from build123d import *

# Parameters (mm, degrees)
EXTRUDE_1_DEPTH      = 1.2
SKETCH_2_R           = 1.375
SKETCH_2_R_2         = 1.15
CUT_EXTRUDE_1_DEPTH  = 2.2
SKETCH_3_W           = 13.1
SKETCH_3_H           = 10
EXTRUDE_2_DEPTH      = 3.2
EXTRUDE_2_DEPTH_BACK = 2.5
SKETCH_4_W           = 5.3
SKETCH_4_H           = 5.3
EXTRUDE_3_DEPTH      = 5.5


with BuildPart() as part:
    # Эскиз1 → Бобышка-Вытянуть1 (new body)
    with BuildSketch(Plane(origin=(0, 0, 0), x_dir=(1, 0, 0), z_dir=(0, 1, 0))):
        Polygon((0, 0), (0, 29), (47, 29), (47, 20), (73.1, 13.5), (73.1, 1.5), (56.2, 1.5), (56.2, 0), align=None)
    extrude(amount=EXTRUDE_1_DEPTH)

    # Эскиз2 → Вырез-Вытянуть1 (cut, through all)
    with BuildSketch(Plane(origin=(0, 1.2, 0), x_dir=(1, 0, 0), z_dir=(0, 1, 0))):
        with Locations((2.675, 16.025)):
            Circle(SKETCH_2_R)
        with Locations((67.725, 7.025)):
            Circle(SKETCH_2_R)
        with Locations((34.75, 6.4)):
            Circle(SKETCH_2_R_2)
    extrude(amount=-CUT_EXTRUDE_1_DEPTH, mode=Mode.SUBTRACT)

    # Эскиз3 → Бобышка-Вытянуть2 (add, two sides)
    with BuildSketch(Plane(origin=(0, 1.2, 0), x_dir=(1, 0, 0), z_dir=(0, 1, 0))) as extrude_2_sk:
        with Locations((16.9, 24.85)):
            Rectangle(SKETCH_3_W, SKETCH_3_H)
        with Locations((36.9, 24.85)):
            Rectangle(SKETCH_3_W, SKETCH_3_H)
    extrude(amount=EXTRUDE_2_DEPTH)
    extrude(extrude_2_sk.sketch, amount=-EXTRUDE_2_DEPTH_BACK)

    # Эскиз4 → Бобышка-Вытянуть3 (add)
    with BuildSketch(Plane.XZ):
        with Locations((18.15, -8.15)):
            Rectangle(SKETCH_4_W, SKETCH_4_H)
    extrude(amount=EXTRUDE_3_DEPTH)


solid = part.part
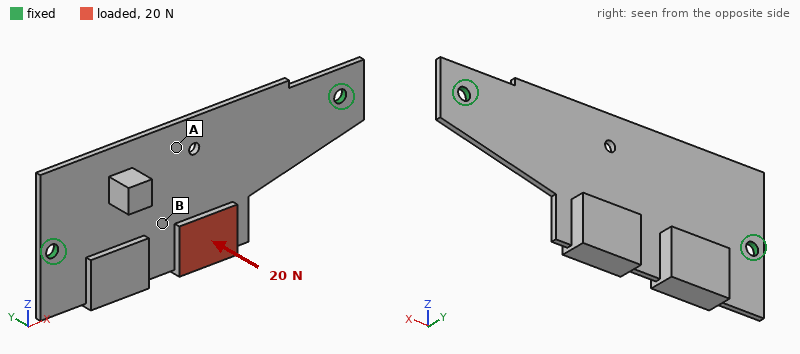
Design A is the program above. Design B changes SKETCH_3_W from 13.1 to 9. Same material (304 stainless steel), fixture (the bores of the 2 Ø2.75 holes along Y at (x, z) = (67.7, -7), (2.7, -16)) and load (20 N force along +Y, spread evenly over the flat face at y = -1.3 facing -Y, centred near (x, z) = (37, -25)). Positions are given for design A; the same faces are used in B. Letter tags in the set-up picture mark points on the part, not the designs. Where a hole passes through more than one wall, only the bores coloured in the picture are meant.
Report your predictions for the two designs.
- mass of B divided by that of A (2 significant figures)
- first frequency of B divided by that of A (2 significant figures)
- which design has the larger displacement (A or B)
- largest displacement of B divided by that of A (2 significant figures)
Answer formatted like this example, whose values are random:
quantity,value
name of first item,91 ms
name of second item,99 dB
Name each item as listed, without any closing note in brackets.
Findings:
quantity,value
mass of B divided by that of A,0.89
first frequency of B divided by that of A,1.1
which design has the larger displacement,B
largest displacement of B divided by that of A,1.1
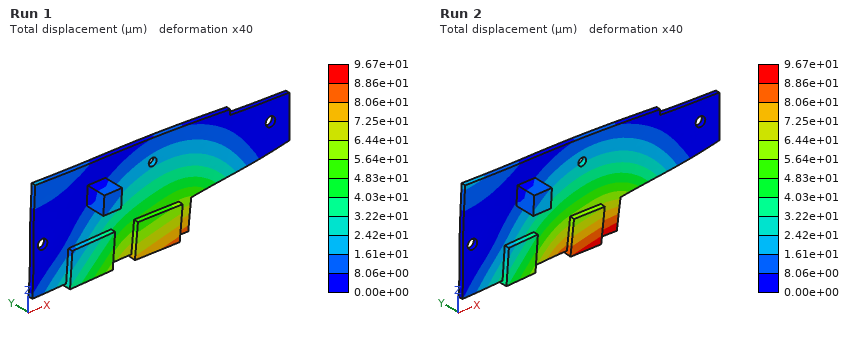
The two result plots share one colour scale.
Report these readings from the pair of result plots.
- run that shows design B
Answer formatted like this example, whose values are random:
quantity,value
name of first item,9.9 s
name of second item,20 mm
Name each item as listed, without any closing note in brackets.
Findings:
quantity,value
run that shows design B,Run 2
